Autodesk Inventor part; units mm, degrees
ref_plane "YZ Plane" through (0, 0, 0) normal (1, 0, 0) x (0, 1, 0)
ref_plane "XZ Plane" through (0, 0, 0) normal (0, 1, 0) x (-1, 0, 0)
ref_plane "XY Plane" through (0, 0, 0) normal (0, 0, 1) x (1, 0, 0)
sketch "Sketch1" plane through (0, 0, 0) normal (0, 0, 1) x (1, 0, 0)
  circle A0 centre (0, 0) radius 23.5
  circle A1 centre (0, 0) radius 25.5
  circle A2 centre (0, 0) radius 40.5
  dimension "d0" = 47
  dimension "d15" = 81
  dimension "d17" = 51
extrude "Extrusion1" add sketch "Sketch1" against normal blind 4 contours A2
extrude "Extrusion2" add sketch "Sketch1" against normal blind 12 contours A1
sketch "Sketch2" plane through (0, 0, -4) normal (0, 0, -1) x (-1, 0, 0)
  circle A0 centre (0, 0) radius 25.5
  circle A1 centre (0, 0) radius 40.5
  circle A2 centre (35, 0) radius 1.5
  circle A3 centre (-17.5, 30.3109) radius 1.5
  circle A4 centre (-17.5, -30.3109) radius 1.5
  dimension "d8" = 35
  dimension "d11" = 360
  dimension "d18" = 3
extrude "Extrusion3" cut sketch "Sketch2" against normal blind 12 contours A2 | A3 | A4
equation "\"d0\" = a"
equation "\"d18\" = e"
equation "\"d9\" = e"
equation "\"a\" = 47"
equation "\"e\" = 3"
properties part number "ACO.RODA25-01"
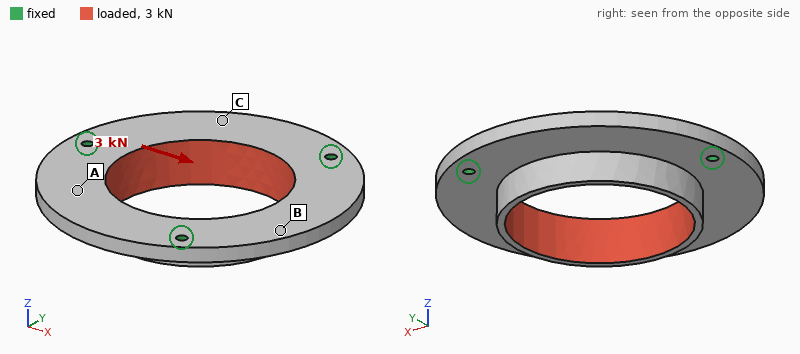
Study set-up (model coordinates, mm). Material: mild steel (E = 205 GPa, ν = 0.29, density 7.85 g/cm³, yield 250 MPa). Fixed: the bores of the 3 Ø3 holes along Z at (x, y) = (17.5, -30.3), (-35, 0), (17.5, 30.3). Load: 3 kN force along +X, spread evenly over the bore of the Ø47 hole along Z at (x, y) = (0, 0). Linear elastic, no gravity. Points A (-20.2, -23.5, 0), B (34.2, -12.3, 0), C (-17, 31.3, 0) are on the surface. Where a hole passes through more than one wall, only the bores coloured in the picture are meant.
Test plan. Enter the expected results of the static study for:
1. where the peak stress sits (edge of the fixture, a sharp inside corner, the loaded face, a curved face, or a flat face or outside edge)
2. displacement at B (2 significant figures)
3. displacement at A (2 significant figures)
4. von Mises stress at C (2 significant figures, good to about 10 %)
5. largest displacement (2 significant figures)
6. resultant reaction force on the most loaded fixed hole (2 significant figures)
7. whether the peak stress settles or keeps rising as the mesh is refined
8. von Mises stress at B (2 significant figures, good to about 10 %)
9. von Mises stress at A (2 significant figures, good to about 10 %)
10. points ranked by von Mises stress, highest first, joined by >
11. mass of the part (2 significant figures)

edge of the fixture
11 µm
5.1 µm
8.1 MPa
16 µm
1.2 kN
keeps rising
15 MPa
4.5 MPa
B > C > A
130 g
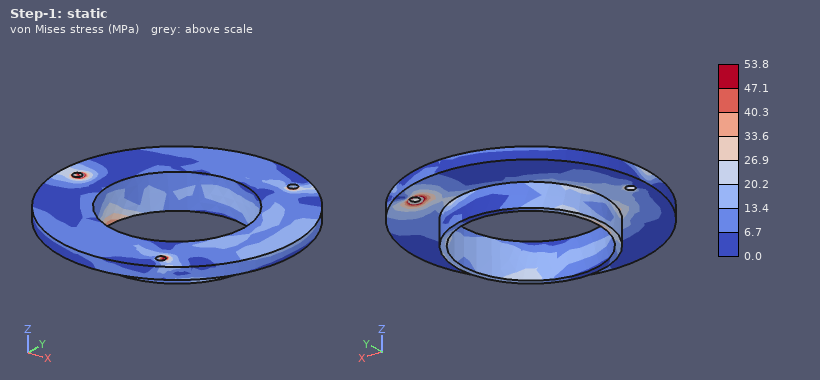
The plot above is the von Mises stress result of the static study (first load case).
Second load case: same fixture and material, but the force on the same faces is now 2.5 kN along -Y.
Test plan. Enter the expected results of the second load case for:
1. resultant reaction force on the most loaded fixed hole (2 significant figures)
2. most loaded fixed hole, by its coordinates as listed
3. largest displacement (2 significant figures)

1.1 kN
(-35, 0)
12 µm
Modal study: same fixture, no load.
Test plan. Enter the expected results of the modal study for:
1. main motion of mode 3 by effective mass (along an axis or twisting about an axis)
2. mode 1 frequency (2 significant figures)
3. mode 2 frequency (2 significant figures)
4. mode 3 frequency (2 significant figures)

along Z
3800 Hz
3800 Hz
4900 Hz
